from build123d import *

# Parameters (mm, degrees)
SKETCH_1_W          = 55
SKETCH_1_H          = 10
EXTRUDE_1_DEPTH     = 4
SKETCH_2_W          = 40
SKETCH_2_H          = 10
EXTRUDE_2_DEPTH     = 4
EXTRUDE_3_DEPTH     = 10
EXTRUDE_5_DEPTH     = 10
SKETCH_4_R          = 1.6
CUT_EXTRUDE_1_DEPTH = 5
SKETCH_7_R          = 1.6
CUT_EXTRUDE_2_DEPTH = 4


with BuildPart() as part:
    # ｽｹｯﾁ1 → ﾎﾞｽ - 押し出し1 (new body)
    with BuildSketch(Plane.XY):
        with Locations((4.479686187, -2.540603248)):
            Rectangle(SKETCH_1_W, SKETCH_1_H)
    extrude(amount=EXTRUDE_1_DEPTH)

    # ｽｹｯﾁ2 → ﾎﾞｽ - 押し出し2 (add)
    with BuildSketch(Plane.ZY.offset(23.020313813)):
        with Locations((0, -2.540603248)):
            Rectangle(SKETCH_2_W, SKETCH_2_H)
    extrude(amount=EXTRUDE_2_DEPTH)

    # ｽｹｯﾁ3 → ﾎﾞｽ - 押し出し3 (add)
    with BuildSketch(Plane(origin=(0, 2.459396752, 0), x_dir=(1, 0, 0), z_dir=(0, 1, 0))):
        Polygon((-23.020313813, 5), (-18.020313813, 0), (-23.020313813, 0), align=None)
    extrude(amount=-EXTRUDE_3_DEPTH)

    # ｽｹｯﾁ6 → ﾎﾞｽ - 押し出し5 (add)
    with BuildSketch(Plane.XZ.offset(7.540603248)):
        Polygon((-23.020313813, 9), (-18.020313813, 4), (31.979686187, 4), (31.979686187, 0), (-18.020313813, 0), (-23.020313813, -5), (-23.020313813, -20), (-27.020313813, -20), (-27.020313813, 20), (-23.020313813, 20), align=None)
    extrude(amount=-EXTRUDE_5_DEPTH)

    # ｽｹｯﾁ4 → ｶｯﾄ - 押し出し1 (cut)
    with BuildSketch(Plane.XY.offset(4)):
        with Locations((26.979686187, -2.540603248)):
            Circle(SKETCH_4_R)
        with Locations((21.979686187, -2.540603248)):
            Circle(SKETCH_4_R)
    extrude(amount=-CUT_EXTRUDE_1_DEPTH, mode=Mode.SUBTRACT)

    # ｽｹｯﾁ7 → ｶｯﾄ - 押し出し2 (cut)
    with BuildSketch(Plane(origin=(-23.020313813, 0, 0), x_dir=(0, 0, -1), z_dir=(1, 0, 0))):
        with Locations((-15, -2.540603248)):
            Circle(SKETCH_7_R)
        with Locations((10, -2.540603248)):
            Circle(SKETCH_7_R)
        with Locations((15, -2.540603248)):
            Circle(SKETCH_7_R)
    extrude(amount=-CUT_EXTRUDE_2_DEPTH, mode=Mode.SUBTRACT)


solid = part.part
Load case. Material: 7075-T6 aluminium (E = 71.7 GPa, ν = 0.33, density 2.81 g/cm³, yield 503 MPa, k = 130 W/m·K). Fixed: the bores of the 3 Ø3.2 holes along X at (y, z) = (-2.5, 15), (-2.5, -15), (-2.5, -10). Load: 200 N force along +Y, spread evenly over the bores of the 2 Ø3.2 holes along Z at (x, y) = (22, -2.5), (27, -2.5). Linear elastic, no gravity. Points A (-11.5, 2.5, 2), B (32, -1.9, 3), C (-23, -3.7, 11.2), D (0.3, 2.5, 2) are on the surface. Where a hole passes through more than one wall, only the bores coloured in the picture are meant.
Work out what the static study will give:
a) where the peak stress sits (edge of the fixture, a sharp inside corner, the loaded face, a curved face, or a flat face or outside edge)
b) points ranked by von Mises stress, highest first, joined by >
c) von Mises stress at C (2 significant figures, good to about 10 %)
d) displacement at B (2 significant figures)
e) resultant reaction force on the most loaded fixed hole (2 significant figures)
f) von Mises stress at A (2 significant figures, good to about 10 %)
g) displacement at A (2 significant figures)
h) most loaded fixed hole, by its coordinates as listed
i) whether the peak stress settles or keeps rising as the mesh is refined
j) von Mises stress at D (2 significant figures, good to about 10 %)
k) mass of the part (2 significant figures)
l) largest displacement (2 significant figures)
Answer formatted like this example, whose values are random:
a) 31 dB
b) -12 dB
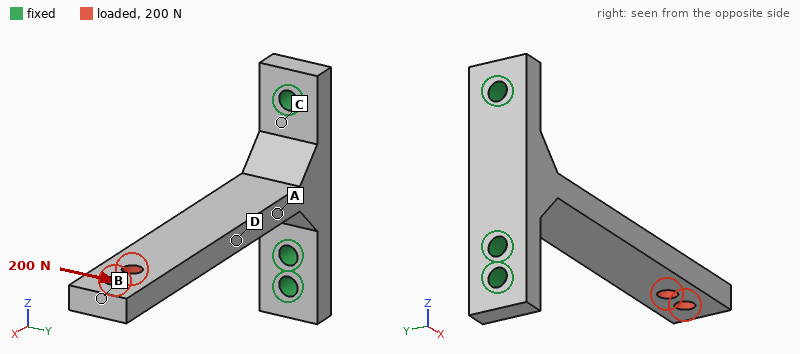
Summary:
a) edge of the fixture
b) C > A > D > B
c) 130 MPa
d) 0.73 mm
e) 250 N
f) 110 MPa
g) 0.12 mm
h) (-2.5, -10)
i) keeps rising
j) 73 MPa
k) 11 g
l) 0.73 mm
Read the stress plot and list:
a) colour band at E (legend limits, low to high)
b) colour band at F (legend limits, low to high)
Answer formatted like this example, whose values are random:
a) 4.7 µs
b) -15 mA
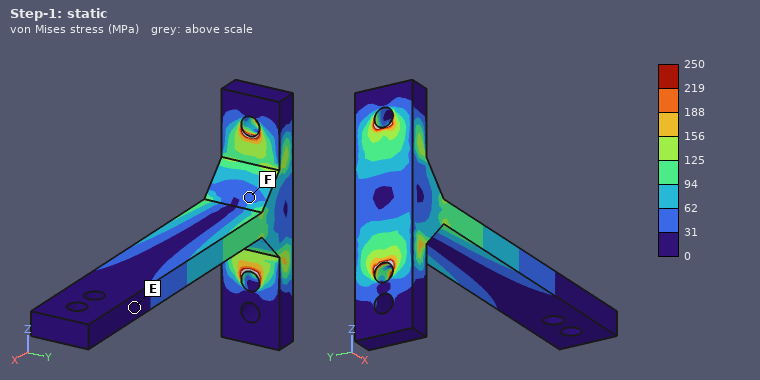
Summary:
a) 0 to 31 MPa
b) 31 to 62 MPa
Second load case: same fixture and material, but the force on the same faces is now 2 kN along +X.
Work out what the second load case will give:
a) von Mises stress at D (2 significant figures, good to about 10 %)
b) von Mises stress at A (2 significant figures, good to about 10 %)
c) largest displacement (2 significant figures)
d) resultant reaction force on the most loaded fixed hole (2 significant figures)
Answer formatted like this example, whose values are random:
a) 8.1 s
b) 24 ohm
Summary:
a) 50 MPa
b) 50 MPa
c) 55 µm
d) 1.2 kN
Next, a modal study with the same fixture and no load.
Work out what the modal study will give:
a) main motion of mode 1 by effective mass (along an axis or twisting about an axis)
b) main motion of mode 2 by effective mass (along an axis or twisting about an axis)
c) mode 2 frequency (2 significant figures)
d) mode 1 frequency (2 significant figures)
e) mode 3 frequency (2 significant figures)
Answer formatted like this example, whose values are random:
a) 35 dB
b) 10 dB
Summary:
a) along Z
b) along Y
c) 1900 Hz
d) 1300 Hz
e) 7300 Hz
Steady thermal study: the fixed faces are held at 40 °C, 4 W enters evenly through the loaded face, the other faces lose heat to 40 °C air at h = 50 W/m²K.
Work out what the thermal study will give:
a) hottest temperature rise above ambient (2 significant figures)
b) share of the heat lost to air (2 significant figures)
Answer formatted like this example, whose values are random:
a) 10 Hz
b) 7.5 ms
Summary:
a) 30 K
b) 33 %
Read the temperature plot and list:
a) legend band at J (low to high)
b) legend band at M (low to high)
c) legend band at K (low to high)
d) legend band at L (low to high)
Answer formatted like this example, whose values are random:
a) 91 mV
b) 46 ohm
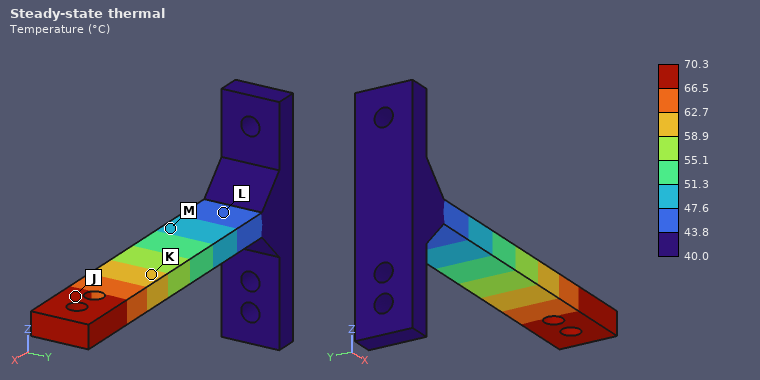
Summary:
a) 66.5 to 70.3 °C
b) 47.6 to 51.3 °C
c) 58.9 to 62.7 °C
d) 43.8 to 47.6 °C
